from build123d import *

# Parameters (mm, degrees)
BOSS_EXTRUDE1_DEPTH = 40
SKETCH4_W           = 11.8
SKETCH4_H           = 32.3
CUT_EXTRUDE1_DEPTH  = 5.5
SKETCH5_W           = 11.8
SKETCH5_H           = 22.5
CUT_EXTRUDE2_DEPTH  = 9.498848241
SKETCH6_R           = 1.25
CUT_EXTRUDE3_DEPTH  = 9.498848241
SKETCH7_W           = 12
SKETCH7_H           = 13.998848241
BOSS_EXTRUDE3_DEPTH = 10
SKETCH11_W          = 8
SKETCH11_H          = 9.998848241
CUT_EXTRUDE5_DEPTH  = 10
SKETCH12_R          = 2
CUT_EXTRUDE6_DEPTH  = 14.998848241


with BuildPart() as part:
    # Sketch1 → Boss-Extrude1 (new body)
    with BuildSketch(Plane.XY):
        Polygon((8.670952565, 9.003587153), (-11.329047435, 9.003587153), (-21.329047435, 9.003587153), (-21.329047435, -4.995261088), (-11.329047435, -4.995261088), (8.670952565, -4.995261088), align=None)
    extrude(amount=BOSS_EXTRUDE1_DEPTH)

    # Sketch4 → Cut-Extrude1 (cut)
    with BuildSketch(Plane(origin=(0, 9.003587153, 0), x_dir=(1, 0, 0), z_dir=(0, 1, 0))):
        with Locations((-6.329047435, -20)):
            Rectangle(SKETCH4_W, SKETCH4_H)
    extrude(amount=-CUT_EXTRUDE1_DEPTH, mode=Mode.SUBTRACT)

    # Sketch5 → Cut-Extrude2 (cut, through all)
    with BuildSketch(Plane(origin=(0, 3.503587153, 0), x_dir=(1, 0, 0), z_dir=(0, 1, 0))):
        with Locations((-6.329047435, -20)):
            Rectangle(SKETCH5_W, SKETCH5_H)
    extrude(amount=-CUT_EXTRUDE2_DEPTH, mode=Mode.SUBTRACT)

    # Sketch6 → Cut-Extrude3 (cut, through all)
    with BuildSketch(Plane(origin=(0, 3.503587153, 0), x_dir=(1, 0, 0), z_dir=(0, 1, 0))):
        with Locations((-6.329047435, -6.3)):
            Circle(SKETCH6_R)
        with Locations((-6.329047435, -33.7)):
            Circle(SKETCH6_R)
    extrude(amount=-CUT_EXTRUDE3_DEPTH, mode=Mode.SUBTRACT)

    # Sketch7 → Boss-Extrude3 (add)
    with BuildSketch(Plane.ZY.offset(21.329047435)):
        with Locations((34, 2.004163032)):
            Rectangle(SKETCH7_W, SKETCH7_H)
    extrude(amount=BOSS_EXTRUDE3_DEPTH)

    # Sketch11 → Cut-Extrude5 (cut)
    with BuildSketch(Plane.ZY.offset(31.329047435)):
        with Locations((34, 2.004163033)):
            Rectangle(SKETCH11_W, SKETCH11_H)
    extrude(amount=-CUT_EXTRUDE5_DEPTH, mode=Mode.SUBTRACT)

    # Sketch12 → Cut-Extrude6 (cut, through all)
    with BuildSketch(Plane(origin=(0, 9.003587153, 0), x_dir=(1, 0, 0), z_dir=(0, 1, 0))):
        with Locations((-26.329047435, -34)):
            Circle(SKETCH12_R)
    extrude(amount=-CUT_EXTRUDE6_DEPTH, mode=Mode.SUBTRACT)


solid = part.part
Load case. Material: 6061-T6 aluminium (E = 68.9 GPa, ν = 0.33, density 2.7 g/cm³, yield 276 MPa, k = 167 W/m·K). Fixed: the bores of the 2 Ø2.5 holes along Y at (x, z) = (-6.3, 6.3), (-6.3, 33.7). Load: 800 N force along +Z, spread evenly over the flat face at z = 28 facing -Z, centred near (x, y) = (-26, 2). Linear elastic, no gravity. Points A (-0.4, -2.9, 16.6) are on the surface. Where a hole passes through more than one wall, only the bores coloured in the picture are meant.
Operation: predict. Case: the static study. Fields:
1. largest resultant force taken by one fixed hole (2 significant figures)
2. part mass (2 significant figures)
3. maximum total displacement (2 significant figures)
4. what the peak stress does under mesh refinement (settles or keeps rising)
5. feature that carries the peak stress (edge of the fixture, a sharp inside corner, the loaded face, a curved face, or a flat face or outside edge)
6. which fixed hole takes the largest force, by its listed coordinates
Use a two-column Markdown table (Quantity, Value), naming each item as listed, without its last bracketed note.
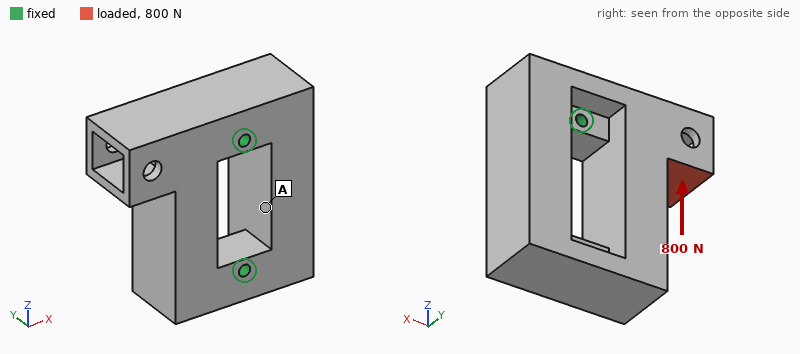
| Quantity | Value |
|---|---|
| largest resultant force taken by one fixed hole | 720 N |
| part mass | 36 g |
| maximum total displacement | 38 µm |
| what the peak stress does under mesh refinement | keeps rising |
| feature that carries the peak stress | edge of the fixture |
| which fixed hole takes the largest force, by its listed coordinates | (-6.3, 6.3) |
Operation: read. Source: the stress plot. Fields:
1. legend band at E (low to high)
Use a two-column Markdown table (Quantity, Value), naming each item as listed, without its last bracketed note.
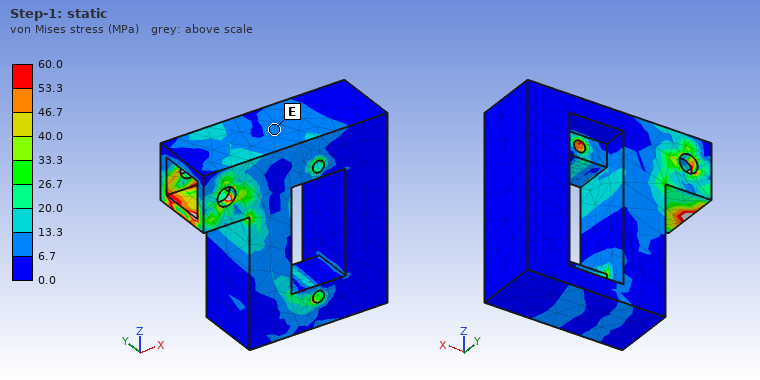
| Quantity | Value |
|---|---|
| legend band at E | 6.7 to 13.3 MPa |
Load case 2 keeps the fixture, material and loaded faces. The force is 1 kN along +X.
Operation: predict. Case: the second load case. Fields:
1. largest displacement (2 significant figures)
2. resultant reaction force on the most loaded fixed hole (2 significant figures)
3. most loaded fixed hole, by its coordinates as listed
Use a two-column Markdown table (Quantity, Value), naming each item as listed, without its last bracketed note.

| Quantity | Value |
|---|---|
| largest displacement | 20 µm |
| resultant reaction force on the most loaded fixed hole | 830 N |
| most loaded fixed hole, by its coordinates as listed | (-6.3, 33.7) |
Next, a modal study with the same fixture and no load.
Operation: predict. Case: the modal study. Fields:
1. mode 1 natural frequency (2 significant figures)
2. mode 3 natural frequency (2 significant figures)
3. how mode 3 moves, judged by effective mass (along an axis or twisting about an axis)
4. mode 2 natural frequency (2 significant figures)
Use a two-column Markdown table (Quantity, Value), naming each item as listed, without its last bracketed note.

| Quantity | Value |
|---|---|
| mode 1 natural frequency | 9400 Hz |
| mode 3 natural frequency | 15 kHz |
| how mode 3 moves, judged by effective mass | along Y |
| mode 2 natural frequency | 14 kHz |
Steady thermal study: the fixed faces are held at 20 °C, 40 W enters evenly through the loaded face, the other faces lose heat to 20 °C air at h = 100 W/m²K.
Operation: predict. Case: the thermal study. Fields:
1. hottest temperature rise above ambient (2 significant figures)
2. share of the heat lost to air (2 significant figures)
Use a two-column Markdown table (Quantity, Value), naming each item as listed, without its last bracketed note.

| Quantity | Value |
|---|---|
| hottest temperature rise above ambient | 53 K |
| share of the heat lost to air | 13 % |
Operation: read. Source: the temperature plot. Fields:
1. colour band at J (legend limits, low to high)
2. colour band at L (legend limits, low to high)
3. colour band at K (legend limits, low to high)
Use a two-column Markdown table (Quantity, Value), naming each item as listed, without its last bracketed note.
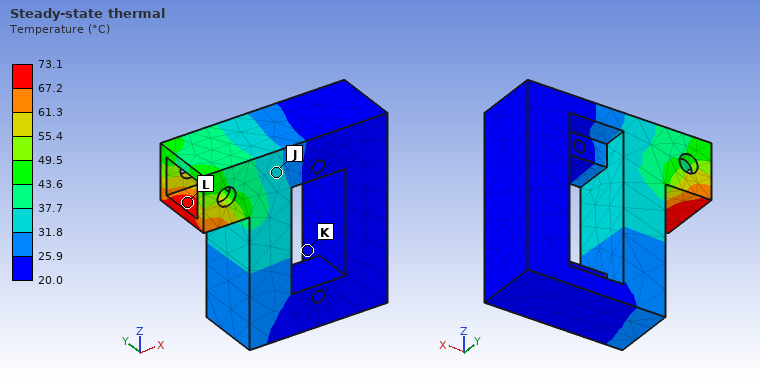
| Quantity | Value |
|---|---|
| colour band at J | 31.8 to 37.7 °C |
| colour band at L | 67.2 to 73.1 °C |
| colour band at K | 20.0 to 25.9 °C |
